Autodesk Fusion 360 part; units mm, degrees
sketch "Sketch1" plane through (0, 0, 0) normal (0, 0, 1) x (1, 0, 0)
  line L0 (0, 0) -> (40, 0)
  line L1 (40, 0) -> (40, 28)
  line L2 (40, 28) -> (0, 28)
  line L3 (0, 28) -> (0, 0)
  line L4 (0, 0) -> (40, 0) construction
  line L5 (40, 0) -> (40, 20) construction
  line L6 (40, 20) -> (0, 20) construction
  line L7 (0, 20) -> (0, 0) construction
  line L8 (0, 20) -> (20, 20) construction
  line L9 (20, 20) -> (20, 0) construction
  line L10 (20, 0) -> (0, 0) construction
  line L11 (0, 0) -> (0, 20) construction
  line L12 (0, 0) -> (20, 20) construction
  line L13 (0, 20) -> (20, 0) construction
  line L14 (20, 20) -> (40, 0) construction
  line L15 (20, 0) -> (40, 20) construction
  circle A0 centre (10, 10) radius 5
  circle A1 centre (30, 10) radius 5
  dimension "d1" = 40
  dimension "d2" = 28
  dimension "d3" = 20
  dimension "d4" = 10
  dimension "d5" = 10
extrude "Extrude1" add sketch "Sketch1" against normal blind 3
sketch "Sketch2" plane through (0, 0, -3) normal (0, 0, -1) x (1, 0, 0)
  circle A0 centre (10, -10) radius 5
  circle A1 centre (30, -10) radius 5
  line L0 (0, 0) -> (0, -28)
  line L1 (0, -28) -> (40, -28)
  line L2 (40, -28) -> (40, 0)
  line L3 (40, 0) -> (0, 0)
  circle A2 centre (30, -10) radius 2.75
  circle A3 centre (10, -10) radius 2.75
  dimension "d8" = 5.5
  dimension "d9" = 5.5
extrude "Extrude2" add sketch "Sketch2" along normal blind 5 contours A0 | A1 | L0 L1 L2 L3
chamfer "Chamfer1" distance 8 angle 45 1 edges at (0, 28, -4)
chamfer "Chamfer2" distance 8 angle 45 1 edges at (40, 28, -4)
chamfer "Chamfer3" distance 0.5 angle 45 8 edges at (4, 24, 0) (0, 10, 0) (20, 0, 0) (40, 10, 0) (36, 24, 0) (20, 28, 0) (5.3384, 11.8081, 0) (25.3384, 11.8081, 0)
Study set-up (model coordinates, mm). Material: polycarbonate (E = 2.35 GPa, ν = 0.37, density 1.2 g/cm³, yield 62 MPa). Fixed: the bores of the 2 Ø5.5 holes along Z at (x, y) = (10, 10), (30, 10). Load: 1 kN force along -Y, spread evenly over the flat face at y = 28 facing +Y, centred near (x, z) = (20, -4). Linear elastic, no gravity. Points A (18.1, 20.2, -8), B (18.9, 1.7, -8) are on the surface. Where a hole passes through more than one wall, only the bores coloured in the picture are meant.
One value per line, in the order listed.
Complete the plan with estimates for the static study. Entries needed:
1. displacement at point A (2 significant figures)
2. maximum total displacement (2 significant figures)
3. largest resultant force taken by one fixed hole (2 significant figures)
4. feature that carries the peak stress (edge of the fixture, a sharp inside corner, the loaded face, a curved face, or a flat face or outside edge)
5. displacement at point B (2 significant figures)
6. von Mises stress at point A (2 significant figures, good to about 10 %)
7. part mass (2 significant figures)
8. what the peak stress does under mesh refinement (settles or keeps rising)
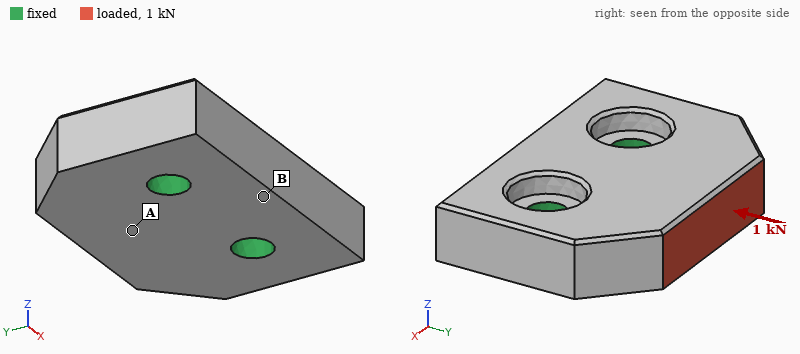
33 µm
77 µm
520 N
edge of the fixture
16 µm
4.9 MPa
9.3 g
keeps rising
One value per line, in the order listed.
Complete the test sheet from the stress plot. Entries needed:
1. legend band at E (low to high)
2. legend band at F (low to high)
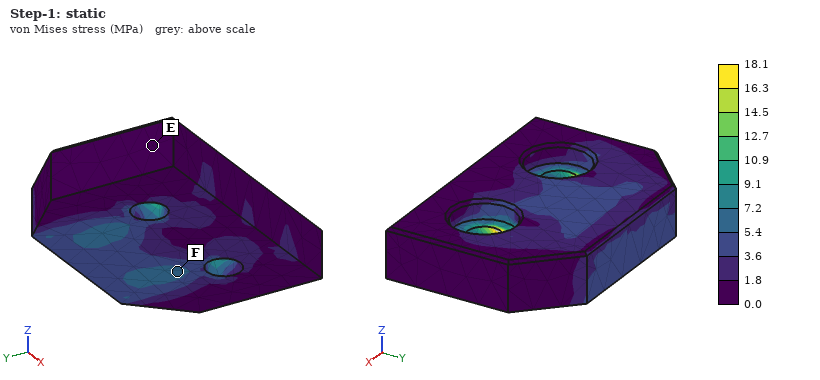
0.0 to 1.8 MPa
5.4 to 7.2 MPa
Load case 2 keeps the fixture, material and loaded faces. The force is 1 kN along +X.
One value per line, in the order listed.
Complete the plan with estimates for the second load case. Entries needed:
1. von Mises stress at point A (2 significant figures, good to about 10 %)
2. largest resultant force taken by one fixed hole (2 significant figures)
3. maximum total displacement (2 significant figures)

12 MPa
890 N
0.15 mm
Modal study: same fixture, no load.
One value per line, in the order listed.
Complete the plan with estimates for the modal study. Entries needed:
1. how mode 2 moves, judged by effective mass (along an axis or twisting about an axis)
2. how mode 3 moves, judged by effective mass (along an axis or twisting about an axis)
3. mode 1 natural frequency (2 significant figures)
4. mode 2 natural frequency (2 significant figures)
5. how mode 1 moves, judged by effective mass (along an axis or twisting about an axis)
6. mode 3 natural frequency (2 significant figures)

twisting about Y
along X
3900 Hz
6500 Hz
along Z
8400 Hz
